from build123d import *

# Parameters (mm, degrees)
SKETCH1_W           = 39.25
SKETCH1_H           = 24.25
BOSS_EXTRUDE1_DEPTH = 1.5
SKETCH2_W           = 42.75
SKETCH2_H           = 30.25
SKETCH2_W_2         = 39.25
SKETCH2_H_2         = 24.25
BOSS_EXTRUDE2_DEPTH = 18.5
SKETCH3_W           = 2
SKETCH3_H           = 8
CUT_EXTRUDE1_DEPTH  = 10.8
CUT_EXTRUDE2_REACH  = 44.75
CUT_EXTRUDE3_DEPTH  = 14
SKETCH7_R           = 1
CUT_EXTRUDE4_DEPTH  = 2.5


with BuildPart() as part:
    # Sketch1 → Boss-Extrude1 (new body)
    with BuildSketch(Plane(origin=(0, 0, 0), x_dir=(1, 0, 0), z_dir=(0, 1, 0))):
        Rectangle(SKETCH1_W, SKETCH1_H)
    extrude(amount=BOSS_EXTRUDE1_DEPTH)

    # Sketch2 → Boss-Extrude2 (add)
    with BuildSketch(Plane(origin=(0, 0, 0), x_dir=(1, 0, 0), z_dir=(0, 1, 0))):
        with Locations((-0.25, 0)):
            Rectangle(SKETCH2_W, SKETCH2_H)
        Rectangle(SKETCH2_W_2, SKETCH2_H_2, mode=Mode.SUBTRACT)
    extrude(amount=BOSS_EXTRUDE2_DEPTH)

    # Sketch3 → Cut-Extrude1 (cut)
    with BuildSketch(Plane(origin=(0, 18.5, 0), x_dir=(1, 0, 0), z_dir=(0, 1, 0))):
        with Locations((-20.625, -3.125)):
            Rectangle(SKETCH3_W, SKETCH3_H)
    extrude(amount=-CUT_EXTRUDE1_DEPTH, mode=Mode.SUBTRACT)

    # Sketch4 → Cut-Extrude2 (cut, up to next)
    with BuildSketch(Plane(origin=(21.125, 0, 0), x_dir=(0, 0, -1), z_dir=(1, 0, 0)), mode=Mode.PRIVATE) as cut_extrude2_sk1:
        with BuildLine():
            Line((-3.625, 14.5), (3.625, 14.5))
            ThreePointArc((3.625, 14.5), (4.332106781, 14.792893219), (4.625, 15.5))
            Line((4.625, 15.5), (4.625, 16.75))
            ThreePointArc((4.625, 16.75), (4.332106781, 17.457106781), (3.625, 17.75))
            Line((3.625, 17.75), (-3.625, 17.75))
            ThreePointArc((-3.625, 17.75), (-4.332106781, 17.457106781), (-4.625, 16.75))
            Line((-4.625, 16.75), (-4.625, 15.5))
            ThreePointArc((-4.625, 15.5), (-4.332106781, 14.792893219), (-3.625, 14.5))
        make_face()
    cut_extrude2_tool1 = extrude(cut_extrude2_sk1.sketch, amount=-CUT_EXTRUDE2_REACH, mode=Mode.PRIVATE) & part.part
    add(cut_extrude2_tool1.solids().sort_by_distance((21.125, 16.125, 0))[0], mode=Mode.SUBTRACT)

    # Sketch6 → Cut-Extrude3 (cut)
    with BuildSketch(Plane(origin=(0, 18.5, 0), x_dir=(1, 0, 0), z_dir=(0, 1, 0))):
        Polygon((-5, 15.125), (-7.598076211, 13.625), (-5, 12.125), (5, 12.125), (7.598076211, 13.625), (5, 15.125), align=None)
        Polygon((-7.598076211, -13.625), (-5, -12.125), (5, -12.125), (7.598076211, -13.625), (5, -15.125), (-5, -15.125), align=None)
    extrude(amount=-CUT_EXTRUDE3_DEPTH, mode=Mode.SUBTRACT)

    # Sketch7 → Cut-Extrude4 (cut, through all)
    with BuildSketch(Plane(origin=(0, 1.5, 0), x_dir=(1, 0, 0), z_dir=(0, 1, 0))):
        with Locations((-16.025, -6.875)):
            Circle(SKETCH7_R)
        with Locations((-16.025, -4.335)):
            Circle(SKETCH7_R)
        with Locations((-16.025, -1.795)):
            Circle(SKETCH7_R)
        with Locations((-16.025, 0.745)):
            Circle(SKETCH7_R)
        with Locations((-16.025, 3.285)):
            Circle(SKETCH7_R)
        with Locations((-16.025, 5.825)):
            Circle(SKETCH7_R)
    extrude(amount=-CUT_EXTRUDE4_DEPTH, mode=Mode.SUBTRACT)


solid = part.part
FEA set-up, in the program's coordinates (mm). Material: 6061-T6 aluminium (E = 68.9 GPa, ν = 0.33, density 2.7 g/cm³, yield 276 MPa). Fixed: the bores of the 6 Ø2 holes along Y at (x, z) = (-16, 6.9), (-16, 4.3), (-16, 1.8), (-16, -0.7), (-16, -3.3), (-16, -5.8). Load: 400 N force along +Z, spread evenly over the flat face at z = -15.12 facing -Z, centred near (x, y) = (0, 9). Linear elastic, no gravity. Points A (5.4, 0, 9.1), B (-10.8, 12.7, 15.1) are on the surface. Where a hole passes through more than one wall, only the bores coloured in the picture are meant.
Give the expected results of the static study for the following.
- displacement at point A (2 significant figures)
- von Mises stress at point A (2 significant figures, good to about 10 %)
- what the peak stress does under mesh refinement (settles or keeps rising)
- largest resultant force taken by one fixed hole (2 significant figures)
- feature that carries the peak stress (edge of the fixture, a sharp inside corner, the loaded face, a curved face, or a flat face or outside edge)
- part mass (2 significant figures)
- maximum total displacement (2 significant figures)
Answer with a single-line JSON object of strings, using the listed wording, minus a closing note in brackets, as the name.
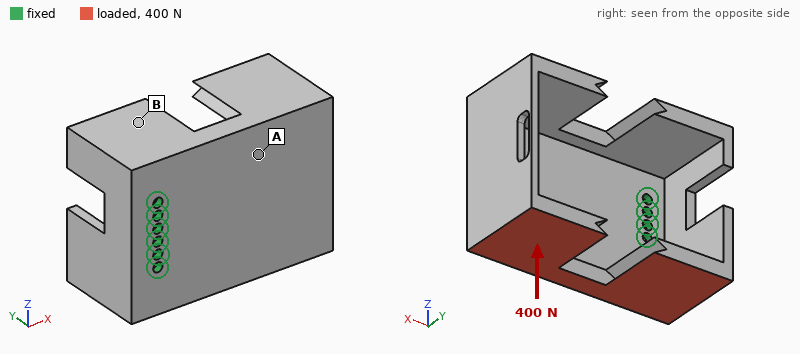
{"displacement at point A": "0.046 mm", "von Mises stress at point A": "22 MPa", "what the peak stress does under mesh refinement": "keeps rising", "largest resultant force taken by one fixed hole": "460 N", "feature that carries the peak stress": "edge of the fixture", "part mass": "17 g", "maximum total displacement": "0.27 mm"}
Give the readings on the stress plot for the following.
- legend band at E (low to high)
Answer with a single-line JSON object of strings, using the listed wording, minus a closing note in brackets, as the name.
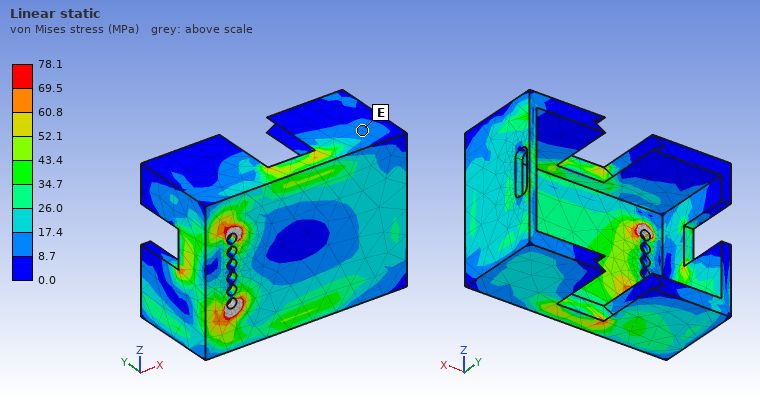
{"legend band at E": "8.7 to 17.4 MPa"}
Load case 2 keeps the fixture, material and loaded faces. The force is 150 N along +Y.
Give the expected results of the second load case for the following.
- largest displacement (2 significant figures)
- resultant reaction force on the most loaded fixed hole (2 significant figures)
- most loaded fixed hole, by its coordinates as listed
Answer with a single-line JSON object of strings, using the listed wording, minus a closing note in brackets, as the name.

{"largest displacement": "0.51 mm", "resultant reaction force on the most loaded fixed hole": "260 N", "most loaded fixed hole, by its coordinates as listed": "(-16, -5.8)"}
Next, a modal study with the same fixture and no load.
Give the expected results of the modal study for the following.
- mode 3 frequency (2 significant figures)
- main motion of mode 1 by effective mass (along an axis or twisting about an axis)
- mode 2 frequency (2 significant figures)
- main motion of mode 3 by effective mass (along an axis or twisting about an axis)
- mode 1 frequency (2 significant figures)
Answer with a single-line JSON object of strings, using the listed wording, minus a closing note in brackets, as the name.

{"mode 3 frequency": "4400 Hz", "main motion of mode 1 by effective mass": "along Y", "mode 2 frequency": "1600 Hz", "main motion of mode 3 by effective mass": "along Z", "mode 1 frequency": "850 Hz"}
